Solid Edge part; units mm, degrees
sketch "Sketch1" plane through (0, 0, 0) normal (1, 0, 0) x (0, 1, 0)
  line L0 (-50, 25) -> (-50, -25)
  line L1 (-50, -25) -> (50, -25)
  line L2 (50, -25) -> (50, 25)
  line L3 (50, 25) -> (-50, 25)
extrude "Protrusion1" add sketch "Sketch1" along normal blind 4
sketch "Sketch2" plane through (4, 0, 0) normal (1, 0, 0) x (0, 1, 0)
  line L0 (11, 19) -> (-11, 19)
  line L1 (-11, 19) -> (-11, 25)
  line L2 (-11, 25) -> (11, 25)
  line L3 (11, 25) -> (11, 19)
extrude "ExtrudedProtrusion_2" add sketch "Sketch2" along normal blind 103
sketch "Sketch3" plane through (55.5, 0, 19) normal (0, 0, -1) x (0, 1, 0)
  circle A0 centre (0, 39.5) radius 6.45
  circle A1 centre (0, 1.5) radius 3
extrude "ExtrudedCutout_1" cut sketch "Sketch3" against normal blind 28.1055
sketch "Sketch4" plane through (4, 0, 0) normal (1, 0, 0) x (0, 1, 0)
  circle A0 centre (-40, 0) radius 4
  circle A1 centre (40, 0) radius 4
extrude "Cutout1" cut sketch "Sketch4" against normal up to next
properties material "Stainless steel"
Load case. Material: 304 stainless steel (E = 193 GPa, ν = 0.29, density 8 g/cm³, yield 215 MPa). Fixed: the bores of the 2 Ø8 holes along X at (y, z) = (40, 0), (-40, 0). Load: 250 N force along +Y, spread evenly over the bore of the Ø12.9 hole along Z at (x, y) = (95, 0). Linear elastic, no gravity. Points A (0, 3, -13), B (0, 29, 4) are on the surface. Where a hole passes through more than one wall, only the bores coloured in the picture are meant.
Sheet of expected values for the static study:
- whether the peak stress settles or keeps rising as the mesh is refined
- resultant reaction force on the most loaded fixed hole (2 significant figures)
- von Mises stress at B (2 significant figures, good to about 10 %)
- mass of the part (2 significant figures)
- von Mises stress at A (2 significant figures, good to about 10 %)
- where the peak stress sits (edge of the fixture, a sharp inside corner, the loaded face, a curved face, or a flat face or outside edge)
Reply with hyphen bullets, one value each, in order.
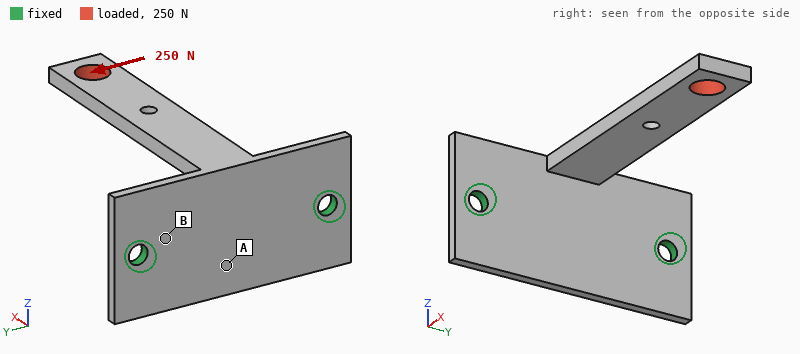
- keeps rising
- 440 N
- 39 MPa
- 260 g
- 15 MPa
- a sharp inside corner
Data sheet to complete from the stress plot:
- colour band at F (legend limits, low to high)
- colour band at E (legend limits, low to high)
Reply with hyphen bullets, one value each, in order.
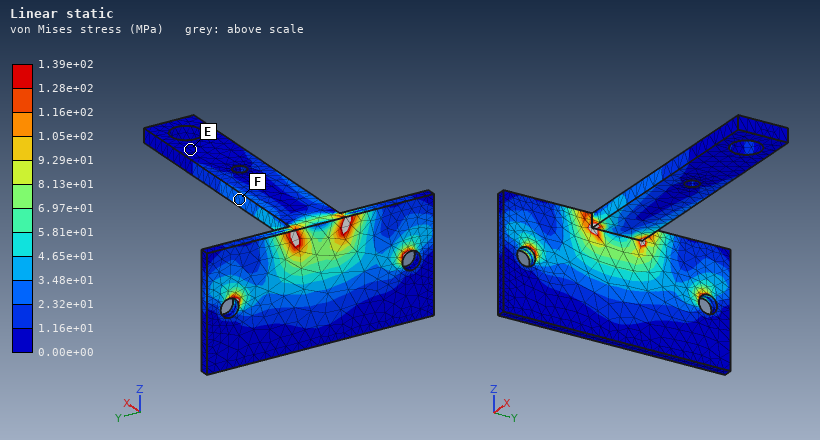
- 2.32e+01 to 3.48e+01 MPa
- 0.00e+00 to 1.16e+01 MPa
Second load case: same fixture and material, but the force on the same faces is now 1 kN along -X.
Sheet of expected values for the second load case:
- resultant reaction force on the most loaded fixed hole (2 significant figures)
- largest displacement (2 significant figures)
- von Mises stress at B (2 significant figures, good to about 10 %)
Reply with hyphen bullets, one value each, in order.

- 510 N
- 0.54 mm
- 85 MPa
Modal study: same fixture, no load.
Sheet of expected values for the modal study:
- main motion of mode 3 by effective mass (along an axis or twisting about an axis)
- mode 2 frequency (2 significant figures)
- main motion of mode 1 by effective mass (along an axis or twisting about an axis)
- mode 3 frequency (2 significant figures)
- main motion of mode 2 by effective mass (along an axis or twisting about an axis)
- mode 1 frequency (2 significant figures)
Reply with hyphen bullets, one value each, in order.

- along X
- 650 Hz
- along Z
- 1400 Hz
- along Y
- 310 Hz
